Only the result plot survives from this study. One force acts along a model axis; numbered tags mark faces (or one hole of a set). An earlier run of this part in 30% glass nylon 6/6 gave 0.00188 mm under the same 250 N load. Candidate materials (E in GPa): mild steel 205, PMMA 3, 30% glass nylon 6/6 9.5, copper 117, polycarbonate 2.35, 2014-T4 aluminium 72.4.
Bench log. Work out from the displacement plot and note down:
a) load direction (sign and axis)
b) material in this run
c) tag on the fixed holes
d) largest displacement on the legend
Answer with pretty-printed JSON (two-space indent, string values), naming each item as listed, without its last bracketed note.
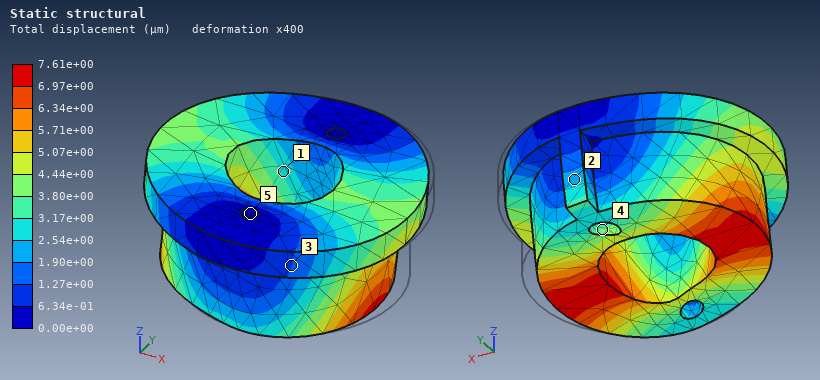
{
  "load direction": "-X",
  "material in this run": "polycarbonate",
  "tag on the fixed holes": "5",
  "largest displacement on the legend": "7.61e+00 µm"
}
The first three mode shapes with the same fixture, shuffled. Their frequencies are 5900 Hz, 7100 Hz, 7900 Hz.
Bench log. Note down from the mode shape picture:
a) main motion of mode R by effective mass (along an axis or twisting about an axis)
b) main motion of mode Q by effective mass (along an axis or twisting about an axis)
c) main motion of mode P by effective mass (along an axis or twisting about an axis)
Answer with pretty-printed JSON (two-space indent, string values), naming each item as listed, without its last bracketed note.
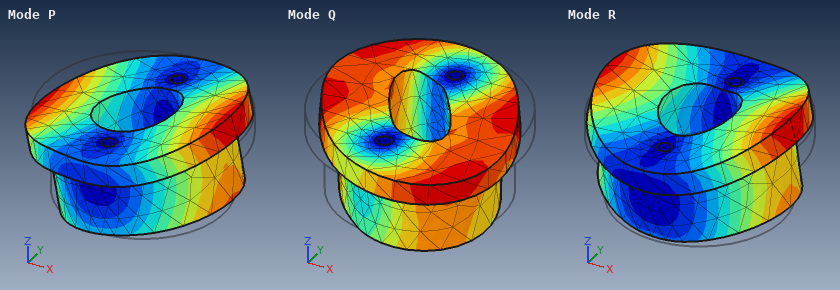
{
  "main motion of mode R by effective mass": "along Z",
  "main motion of mode Q by effective mass": "twisting about Z",
  "main motion of mode P by effective mass": "twisting about Y"
}
